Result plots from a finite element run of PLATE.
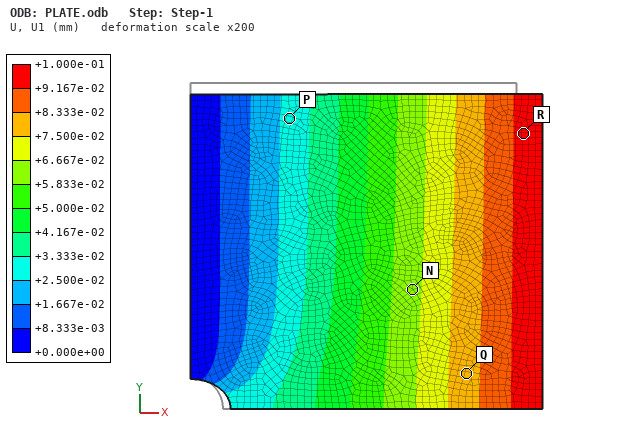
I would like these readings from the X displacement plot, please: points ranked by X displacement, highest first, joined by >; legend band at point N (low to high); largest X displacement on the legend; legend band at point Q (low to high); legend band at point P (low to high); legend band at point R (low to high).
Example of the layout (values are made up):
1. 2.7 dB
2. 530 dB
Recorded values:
1. R > Q > N > P
2. +5.833e-02 to +6.667e-02 mm
3. +1.000e-01 mm
4. +7.500e-02 to +8.333e-02 mm
5. +2.500e-02 to +3.333e-02 mm
6. +9.167e-02 to +1.000e-01 mm
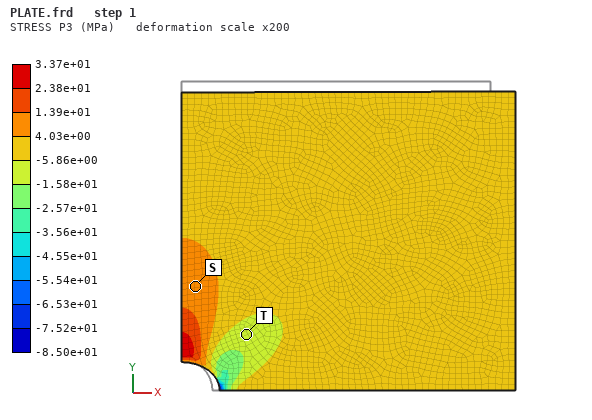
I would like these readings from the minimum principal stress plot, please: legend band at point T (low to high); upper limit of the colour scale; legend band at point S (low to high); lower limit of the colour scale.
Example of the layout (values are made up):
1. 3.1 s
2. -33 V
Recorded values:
1. -1.58e+01 to -5.86e+00 MPa
2. 3.37e+01 MPa
3. 4.03e+00 to 1.39e+01 MPa
4. -8.50e+01 MPa
